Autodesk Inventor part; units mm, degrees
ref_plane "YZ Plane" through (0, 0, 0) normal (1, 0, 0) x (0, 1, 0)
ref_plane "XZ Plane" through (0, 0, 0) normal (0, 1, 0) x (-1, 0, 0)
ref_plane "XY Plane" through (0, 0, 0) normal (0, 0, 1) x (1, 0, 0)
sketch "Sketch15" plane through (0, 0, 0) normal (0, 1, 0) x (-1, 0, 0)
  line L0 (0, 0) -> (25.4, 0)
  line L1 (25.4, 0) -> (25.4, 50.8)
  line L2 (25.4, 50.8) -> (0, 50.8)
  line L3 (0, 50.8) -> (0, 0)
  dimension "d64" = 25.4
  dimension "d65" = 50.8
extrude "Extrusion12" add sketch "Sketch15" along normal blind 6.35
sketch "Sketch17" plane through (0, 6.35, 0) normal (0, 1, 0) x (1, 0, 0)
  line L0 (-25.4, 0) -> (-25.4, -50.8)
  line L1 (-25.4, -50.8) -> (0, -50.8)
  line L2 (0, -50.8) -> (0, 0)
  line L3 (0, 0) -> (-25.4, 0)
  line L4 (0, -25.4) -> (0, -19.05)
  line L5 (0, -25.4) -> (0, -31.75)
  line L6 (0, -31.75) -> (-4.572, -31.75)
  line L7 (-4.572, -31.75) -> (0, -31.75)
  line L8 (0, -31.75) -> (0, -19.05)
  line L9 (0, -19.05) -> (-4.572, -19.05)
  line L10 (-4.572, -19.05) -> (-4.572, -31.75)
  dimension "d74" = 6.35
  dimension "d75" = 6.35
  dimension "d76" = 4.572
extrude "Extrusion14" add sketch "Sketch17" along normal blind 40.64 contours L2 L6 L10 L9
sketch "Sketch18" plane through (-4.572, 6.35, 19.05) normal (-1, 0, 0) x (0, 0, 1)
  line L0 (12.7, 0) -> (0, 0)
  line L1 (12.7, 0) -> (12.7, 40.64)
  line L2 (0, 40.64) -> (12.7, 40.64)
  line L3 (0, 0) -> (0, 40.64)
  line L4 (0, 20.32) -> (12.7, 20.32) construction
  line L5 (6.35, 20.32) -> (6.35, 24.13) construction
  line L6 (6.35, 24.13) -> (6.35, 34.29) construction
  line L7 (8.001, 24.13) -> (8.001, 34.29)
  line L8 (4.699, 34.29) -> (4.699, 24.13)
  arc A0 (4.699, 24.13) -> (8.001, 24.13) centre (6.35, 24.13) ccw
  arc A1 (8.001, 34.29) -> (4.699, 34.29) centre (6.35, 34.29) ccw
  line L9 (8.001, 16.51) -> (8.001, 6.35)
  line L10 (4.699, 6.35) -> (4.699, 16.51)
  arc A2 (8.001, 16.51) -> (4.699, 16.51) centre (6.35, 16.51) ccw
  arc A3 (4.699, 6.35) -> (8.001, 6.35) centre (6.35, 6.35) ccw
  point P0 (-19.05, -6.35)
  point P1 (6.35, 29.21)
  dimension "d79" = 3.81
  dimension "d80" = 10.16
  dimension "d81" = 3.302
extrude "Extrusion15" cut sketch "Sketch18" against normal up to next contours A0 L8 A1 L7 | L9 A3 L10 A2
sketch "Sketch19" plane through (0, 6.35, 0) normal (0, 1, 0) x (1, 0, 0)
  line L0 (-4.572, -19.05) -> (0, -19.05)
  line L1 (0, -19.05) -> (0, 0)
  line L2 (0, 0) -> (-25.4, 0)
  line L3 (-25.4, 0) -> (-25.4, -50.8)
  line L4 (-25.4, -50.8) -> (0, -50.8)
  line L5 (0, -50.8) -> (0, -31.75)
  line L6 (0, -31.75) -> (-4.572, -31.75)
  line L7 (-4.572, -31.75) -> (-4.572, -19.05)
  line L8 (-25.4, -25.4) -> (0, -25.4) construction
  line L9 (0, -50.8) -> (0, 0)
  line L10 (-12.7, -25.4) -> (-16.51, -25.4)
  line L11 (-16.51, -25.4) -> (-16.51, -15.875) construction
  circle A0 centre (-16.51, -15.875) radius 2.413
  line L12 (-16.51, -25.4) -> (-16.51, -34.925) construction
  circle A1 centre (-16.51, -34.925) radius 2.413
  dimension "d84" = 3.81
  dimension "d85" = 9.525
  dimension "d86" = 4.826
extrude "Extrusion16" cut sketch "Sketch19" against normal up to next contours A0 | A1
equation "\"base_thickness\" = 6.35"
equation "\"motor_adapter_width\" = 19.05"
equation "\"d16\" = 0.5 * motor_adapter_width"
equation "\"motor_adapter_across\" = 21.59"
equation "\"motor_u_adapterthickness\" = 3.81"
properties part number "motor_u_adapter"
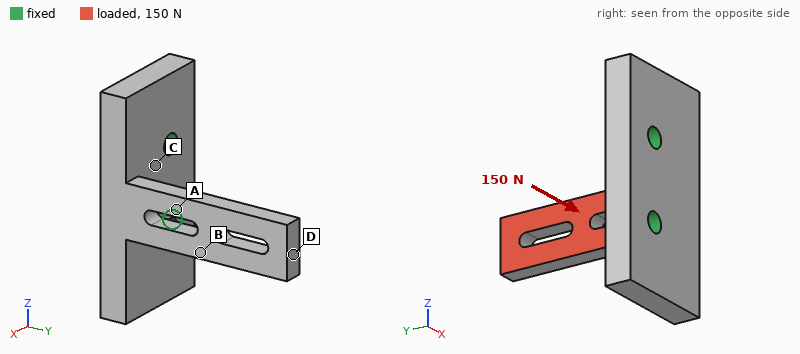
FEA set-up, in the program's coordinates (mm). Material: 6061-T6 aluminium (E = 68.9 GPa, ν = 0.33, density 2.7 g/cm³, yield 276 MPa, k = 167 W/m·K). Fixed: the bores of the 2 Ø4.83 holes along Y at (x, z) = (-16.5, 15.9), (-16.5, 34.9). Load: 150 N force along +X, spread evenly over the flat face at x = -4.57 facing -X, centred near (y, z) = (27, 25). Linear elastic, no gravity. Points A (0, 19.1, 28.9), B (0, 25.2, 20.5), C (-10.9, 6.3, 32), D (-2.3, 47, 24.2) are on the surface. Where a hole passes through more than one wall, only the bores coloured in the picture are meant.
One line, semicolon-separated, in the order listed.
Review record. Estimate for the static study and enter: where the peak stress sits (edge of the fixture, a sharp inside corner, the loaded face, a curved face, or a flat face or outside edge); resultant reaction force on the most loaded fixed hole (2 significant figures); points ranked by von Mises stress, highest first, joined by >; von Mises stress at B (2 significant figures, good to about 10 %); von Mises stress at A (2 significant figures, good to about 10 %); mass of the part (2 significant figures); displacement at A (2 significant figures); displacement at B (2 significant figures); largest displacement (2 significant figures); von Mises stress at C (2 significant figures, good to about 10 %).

the loaded face; 84 N; A > B > C > D; 25 MPa; 44 MPa; 27 g; 0.064 mm; 0.11 mm; 0.30 mm; 16 MPa
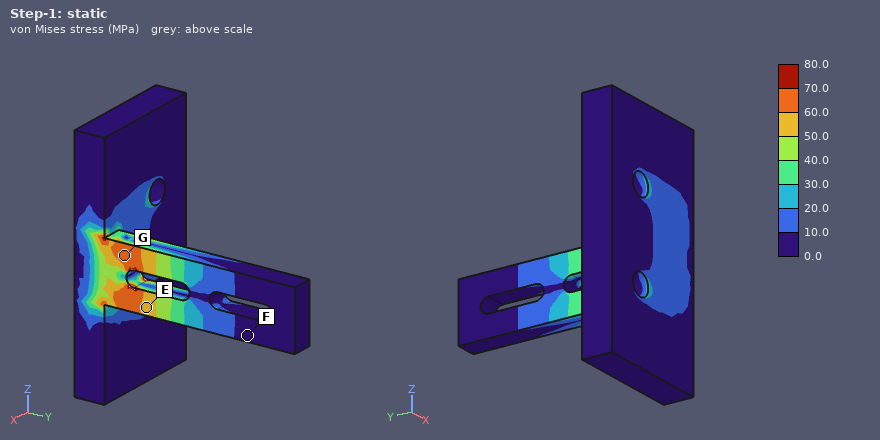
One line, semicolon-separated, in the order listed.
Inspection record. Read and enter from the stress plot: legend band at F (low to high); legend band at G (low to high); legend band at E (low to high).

0.0 to 10.0 MPa; 60.0 to 70.0 MPa; 50.0 to 60.0 MPa
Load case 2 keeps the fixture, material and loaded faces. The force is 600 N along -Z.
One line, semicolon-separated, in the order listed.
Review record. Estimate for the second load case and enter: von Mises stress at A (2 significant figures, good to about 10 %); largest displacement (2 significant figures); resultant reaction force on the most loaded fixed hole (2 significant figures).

31 MPa; 0.27 mm; 770 N
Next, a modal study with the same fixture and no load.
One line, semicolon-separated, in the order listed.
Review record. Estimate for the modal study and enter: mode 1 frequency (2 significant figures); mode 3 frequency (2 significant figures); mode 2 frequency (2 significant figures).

1900 Hz; 9100 Hz; 4000 Hz
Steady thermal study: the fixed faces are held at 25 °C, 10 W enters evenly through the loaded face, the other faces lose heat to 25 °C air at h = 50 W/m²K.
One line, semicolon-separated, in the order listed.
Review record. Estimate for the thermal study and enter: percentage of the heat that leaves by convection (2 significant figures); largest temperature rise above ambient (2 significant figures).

14 %; 28 K
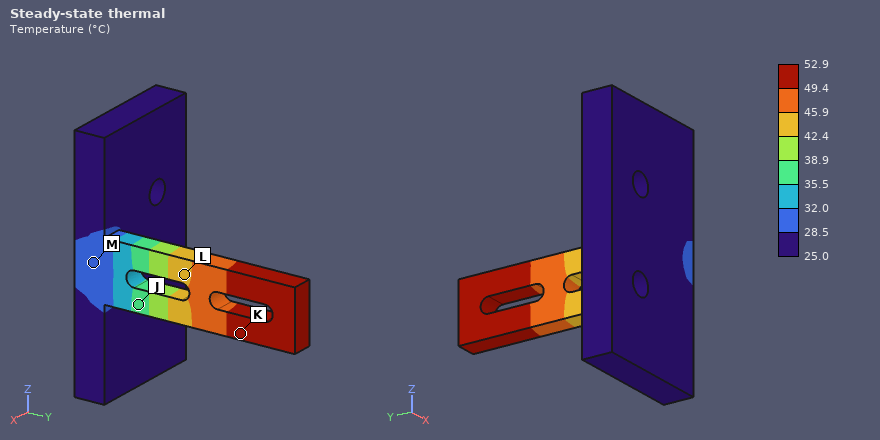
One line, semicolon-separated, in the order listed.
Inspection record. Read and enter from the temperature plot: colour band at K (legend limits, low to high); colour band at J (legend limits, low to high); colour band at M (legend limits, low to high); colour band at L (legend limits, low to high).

49.4 to 52.9 °C; 35.5 to 38.9 °C; 28.5 to 32.0 °C; 42.4 to 45.9 °C
